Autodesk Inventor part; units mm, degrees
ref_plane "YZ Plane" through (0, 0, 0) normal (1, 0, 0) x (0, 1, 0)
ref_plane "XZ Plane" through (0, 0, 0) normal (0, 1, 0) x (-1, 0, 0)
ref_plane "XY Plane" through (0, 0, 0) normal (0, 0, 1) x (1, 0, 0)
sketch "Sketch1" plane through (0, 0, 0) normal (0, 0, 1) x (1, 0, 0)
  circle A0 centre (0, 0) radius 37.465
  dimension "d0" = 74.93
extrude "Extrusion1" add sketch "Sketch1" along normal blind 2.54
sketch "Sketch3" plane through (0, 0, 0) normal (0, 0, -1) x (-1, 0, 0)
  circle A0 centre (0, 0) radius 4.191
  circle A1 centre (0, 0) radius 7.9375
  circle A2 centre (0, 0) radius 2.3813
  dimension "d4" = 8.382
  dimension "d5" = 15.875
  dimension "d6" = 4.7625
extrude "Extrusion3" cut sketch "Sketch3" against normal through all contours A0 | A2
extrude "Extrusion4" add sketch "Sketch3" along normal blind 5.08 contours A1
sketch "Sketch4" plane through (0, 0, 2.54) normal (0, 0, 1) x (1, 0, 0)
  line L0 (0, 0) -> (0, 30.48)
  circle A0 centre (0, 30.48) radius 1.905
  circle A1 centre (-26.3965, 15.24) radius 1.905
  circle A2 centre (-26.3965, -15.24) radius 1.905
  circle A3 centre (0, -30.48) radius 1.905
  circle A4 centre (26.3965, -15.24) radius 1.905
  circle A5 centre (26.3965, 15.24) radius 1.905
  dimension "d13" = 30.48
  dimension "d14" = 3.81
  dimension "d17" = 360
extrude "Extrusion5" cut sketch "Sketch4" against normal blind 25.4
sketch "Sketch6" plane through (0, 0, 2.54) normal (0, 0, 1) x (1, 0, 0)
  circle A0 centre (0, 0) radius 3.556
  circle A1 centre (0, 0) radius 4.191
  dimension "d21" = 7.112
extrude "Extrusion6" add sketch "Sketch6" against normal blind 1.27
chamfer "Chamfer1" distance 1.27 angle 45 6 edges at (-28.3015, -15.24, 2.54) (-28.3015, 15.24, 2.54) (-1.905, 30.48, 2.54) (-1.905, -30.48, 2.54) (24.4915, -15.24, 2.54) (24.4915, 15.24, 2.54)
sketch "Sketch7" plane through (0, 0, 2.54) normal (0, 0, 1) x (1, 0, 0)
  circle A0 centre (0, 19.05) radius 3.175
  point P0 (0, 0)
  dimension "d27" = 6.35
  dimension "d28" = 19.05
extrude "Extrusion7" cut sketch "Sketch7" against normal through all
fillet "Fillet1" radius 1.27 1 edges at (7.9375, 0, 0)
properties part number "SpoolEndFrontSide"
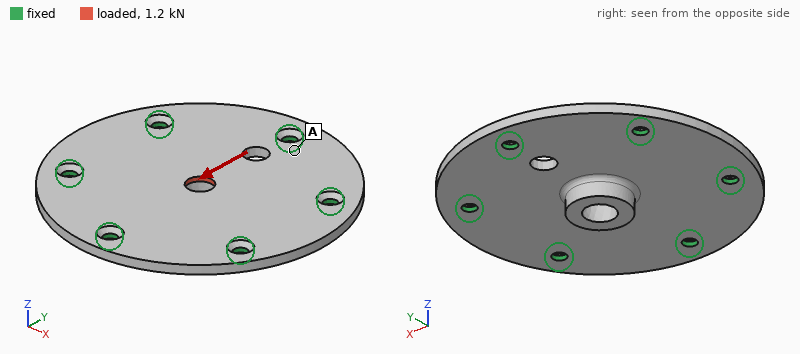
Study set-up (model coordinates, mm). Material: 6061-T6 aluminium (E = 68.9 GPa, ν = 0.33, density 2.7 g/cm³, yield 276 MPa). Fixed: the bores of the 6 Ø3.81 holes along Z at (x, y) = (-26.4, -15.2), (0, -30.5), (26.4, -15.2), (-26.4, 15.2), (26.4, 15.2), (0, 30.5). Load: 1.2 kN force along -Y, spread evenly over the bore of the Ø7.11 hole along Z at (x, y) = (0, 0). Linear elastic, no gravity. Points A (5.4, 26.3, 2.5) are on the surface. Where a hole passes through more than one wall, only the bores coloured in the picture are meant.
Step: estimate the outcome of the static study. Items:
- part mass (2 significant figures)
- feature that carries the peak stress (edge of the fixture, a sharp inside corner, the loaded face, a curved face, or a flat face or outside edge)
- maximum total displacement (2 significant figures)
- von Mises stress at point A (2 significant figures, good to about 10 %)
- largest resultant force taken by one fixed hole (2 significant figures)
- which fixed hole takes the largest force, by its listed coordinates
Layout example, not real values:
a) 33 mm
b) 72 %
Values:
a) 31 g
b) the loaded face
c) 6.4 µm
d) 6.0 MPa
e) 310 N
f) (0, -30.5)
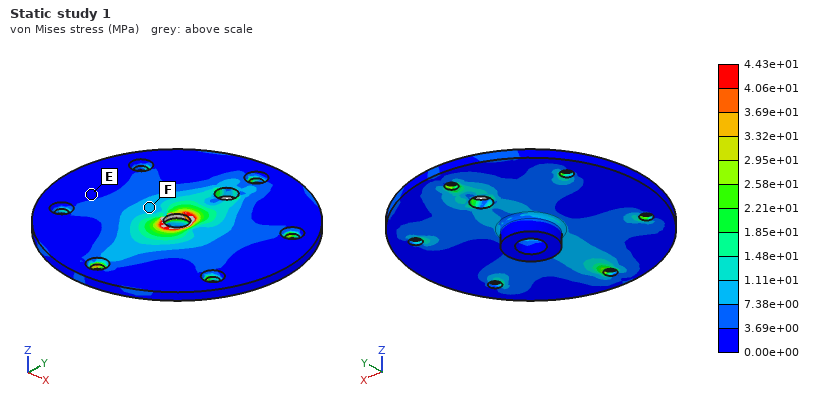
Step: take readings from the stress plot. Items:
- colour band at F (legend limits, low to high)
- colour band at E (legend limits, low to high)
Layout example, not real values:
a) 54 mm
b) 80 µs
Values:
a) 7.38e+00 to 1.11e+01 MPa
b) 0.00e+00 to 3.69e+00 MPa
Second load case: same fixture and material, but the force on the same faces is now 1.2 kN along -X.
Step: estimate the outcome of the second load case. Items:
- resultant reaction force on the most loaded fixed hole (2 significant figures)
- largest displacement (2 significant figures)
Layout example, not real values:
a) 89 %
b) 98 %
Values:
a) 270 N
b) 6.0 µm
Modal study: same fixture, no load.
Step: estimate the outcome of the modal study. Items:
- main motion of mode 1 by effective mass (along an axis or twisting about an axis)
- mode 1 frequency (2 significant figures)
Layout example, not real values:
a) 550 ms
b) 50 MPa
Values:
a) along Z
b) 5200 Hz
